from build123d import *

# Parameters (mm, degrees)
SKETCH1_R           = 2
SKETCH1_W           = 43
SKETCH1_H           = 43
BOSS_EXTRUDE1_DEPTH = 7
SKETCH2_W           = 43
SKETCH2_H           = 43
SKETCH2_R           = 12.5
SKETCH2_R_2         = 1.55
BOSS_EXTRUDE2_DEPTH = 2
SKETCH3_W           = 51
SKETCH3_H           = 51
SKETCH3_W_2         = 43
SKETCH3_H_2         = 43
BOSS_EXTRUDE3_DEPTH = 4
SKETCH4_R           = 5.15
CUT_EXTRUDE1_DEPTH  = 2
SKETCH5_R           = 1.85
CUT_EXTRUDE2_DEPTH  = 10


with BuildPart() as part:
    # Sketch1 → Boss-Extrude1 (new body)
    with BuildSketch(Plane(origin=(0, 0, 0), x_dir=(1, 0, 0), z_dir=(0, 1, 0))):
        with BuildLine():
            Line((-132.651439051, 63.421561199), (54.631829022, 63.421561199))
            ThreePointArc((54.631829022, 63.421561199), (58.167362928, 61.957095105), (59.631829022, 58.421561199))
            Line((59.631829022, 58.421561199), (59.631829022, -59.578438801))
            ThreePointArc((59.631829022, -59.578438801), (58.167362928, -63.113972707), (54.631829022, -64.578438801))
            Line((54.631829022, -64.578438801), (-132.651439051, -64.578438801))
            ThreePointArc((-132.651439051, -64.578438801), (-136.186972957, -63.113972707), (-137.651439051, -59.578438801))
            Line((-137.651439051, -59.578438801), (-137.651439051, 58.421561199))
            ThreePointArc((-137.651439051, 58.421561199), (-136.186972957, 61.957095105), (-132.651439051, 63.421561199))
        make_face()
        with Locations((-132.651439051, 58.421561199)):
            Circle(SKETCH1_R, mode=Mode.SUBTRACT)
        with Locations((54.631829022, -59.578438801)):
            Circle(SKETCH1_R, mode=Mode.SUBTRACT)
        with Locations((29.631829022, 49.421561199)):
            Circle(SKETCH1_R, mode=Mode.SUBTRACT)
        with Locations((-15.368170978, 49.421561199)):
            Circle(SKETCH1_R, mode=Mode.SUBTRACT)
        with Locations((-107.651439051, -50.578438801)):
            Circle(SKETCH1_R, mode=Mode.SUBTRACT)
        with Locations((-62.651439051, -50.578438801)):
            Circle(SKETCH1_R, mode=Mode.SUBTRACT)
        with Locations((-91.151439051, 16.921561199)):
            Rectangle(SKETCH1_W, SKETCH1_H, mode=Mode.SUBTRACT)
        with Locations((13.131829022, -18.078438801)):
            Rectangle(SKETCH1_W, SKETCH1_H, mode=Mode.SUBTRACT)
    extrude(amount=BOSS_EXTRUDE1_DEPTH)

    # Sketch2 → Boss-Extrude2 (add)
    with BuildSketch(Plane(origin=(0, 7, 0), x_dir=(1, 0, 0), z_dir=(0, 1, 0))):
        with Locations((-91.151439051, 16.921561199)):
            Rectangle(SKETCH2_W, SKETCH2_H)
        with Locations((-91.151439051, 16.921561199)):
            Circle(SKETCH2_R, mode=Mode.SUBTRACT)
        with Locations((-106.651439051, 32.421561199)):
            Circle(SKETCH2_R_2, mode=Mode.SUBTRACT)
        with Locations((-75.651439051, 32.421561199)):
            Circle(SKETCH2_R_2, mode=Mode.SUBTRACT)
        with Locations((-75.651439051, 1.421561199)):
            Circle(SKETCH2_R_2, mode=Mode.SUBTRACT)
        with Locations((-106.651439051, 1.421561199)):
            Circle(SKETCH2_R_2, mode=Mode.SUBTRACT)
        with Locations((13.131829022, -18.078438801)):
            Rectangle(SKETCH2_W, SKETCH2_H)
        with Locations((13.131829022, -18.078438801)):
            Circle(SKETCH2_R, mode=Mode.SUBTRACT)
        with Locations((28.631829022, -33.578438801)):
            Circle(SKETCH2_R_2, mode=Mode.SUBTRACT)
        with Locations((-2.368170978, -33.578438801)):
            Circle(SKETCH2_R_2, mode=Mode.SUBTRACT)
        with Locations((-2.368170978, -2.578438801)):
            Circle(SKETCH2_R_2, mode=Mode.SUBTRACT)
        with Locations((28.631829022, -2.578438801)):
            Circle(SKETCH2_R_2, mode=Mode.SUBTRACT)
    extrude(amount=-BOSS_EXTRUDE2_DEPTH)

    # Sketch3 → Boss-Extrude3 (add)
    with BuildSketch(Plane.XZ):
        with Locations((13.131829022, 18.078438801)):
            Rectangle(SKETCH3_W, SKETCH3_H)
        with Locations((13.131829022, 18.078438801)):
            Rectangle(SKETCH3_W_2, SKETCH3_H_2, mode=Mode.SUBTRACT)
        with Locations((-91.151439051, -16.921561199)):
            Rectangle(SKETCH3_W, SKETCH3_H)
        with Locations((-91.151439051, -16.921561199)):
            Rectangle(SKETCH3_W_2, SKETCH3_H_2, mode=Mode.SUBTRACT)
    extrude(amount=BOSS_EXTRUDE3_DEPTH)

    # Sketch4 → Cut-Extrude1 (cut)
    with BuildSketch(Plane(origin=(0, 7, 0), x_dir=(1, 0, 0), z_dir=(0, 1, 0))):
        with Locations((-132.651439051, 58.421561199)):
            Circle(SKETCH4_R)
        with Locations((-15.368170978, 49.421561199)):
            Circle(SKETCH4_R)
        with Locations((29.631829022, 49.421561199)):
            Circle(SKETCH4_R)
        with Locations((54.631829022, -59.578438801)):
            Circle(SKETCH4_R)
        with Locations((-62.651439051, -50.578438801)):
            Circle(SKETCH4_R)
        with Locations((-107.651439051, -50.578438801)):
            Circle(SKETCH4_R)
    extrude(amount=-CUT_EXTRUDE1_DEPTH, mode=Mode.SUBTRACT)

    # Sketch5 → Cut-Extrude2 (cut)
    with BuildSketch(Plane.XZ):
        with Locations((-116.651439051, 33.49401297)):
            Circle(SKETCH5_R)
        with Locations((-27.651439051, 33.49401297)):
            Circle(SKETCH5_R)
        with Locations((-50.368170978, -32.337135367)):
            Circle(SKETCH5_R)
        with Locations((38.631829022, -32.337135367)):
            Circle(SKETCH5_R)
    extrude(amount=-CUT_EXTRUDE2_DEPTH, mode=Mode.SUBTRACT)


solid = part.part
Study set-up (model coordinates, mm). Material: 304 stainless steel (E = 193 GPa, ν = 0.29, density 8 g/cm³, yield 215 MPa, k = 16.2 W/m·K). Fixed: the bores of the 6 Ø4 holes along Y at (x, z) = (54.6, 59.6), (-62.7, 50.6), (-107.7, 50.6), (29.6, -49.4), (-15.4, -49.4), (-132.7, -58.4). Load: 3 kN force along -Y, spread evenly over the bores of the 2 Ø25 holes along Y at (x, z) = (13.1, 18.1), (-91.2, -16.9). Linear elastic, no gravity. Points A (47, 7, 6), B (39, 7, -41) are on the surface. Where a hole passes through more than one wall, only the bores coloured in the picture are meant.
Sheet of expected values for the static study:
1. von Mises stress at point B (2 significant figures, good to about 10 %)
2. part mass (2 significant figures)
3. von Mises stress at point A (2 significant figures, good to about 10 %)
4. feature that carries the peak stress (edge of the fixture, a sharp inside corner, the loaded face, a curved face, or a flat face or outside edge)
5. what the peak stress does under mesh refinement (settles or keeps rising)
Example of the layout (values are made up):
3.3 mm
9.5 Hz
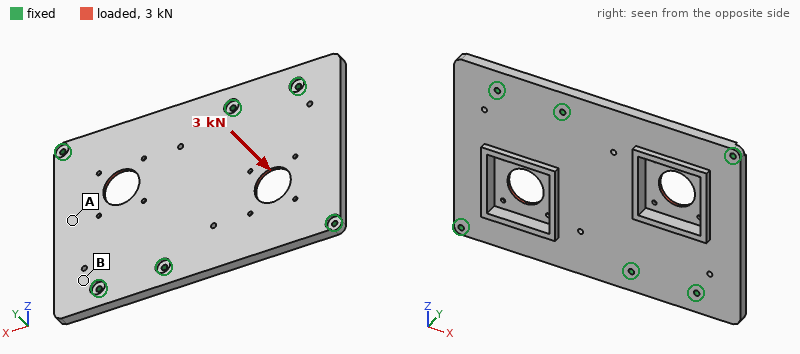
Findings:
14 MPa
1.3 kg
24 MPa
edge of the fixture
keeps rising
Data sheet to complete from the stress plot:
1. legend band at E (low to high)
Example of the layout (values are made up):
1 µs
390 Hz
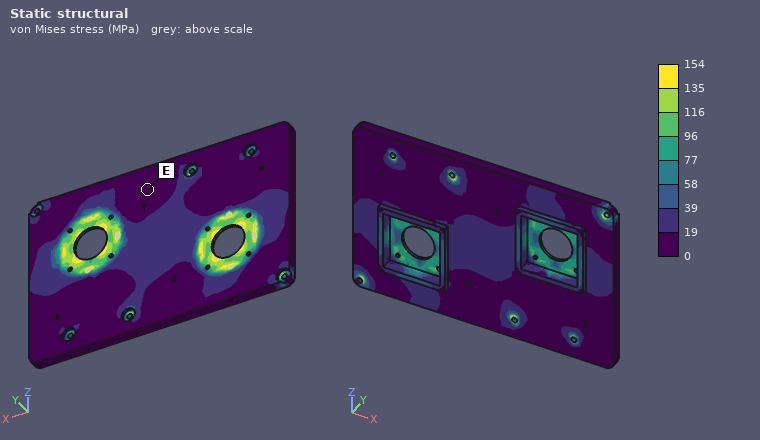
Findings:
0 to 19 MPa
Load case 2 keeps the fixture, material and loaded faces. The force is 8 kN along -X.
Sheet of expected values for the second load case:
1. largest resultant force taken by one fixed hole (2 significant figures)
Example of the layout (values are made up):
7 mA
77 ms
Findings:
1.9 kN
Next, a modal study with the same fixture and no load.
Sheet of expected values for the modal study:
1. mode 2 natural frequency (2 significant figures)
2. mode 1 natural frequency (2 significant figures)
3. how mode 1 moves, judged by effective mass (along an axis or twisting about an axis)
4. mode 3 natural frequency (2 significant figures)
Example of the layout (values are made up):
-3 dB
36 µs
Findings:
2100 Hz
1900 Hz
along Y
2500 Hz
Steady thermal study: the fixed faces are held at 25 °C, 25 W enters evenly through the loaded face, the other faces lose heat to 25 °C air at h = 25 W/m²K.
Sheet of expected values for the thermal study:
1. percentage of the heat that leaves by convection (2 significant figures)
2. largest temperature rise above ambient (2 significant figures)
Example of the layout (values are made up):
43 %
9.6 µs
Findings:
71 %
58 K
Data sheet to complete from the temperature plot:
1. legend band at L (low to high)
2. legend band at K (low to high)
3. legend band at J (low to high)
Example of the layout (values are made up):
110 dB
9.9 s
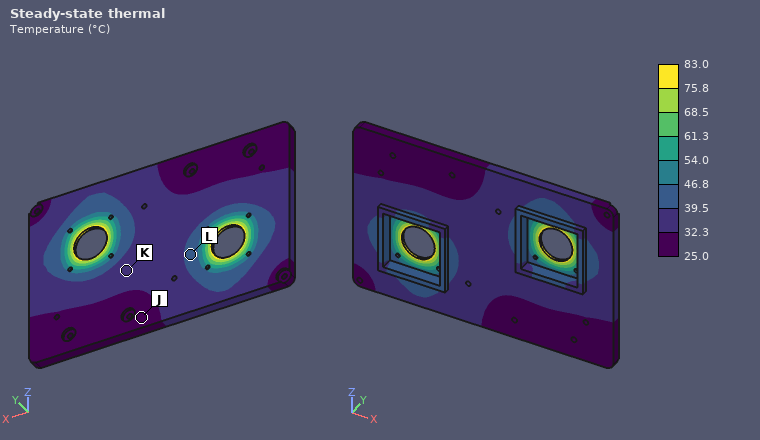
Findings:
39.5 to 46.8 °C
32.3 to 39.5 °C
25.0 to 32.3 °C
